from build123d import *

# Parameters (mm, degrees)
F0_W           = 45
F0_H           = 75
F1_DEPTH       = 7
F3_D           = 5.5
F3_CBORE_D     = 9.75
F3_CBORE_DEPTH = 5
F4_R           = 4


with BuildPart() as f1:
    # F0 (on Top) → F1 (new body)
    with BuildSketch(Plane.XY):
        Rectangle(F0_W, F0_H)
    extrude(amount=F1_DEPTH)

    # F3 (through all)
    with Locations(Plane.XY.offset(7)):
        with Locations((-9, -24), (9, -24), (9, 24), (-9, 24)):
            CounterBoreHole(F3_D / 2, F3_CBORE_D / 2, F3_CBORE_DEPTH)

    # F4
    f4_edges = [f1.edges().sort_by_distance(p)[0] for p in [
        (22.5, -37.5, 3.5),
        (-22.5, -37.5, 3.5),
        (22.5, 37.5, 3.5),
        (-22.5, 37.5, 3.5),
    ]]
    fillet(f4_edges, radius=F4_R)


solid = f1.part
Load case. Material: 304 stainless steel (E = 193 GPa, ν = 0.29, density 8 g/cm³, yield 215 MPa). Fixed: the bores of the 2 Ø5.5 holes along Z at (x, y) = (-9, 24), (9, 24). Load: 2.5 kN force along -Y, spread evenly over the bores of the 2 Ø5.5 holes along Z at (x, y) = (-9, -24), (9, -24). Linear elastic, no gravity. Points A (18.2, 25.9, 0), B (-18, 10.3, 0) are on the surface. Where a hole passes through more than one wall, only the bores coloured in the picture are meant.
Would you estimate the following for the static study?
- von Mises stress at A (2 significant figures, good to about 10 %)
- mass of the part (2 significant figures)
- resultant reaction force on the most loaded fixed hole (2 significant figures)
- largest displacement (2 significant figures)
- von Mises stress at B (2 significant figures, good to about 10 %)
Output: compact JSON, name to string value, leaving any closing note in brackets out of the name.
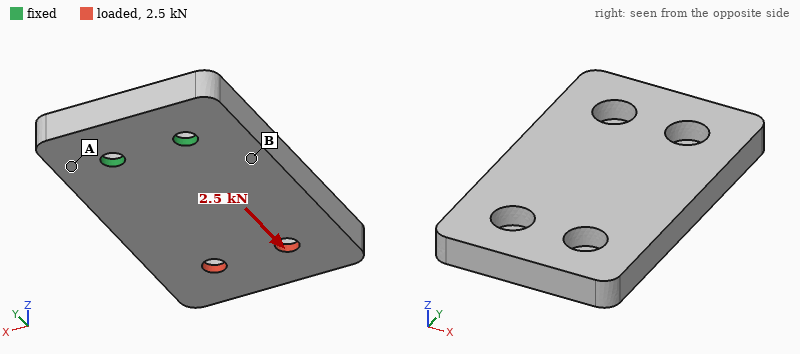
{"von Mises stress at A": "10.0 MPa", "mass of the part": "170 g", "resultant reaction force on the most loaded fixed hole": "1.3 kN", "largest displacement": "38 µm", "von Mises stress at B": "23 MPa"}
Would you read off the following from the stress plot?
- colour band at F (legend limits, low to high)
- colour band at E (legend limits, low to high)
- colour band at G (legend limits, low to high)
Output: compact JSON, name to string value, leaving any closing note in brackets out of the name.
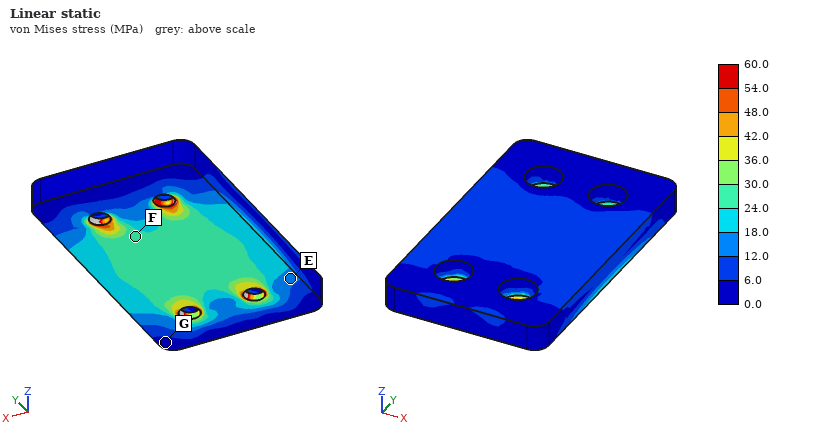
{"colour band at F": "24.0 to 30.0 MPa", "colour band at E": "12.0 to 18.0 MPa", "colour band at G": "0.0 to 6.0 MPa"}
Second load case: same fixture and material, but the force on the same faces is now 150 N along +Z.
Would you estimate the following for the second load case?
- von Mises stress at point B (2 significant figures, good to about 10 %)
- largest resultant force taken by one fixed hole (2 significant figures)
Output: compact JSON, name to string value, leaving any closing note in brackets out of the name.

{"von Mises stress at point B": "14 MPa", "largest resultant force taken by one fixed hole": "95 N"}
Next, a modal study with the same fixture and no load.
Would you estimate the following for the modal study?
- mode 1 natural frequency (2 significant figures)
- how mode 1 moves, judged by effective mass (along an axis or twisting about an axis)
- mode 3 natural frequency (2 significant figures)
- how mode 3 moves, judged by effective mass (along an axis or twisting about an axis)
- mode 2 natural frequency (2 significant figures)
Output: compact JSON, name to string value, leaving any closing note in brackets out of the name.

{"mode 1 natural frequency": "940 Hz", "how mode 1 moves, judged by effective mass": "along Z", "mode 3 natural frequency": "4400 Hz", "how mode 3 moves, judged by effective mass": "along X", "mode 2 natural frequency": "3600 Hz"}
